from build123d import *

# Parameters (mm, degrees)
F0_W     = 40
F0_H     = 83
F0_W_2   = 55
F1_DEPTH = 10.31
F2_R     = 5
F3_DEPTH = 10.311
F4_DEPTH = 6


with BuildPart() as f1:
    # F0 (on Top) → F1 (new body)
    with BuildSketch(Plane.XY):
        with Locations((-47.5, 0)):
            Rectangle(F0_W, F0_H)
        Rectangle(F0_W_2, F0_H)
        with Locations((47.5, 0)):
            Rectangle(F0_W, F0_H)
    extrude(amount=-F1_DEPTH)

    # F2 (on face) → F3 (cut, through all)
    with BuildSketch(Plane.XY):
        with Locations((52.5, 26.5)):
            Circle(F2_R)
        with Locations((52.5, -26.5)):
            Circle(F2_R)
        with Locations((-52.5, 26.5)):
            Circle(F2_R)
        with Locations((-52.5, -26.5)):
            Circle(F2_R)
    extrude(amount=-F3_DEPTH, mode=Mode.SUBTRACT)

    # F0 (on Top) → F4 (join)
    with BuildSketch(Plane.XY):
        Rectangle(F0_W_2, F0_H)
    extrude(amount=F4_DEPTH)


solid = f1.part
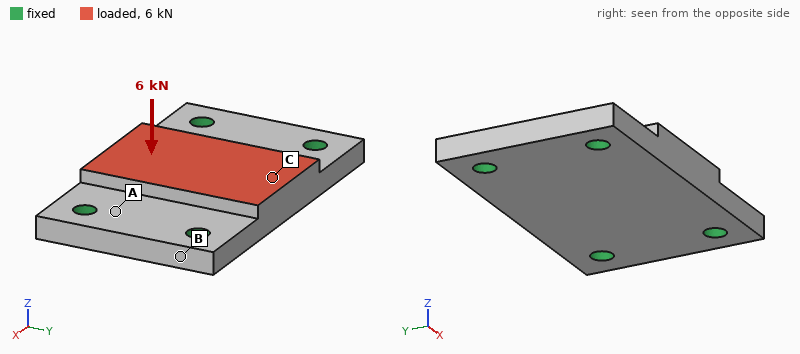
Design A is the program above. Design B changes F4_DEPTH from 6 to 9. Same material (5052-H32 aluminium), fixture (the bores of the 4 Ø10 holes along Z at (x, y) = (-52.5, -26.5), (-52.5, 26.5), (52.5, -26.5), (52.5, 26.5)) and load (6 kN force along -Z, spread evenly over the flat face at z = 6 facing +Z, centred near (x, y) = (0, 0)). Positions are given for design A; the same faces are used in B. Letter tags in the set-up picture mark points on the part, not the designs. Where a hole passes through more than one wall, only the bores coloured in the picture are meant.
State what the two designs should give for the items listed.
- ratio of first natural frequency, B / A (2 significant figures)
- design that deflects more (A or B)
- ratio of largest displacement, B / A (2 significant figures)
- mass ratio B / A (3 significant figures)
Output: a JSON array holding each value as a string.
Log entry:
["1.0", "A", "0.81", "1.10"]
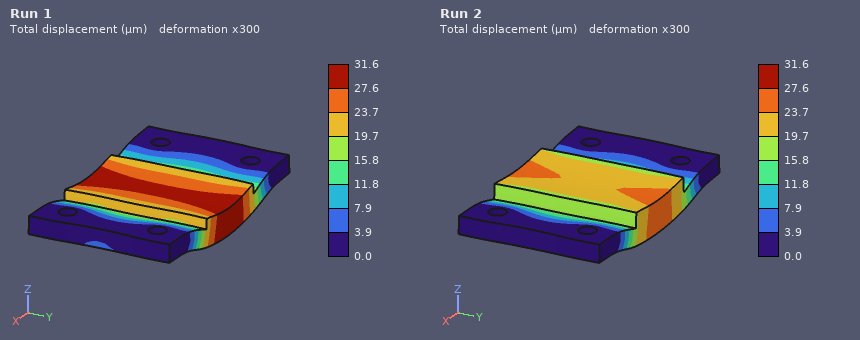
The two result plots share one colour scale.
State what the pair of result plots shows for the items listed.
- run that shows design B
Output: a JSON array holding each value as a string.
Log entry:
["Run 2"]
